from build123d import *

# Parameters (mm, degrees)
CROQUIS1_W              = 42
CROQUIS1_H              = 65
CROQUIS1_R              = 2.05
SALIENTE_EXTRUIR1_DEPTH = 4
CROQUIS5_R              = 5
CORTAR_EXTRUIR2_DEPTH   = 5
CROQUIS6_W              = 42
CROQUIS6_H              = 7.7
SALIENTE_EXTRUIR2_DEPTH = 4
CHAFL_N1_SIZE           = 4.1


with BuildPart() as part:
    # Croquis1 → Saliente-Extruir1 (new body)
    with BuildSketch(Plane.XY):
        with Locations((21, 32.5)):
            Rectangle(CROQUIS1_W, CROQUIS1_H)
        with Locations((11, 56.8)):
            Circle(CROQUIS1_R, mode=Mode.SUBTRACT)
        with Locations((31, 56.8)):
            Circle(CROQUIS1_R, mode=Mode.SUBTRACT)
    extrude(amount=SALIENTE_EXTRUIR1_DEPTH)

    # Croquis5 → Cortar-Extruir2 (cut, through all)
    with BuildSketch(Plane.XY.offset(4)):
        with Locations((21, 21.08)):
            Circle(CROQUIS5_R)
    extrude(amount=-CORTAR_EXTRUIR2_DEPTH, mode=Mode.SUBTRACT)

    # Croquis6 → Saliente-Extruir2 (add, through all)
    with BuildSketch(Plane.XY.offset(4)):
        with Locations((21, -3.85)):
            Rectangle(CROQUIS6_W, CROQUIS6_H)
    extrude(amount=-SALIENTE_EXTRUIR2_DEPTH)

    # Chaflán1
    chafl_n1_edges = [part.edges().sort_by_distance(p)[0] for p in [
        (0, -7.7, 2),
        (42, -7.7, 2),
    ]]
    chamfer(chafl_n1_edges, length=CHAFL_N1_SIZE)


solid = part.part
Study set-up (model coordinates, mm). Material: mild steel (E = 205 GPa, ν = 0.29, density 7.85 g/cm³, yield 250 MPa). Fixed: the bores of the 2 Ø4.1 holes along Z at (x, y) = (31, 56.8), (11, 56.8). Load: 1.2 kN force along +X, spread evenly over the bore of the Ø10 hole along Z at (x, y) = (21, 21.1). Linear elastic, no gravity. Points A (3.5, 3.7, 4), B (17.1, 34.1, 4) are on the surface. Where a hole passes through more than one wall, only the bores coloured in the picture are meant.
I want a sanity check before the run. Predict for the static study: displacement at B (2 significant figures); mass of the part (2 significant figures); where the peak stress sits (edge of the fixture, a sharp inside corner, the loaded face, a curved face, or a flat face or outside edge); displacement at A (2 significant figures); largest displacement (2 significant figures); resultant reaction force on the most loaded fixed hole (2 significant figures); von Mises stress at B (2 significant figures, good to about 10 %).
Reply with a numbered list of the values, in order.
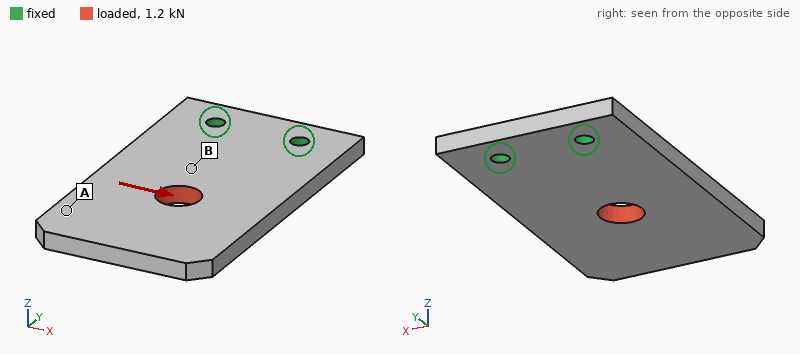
1. 6.4 µm
2. 92 g
3. edge of the fixture
4. 16 µm
5. 19 µm
6. 1.9 kN
7. 20 MPa
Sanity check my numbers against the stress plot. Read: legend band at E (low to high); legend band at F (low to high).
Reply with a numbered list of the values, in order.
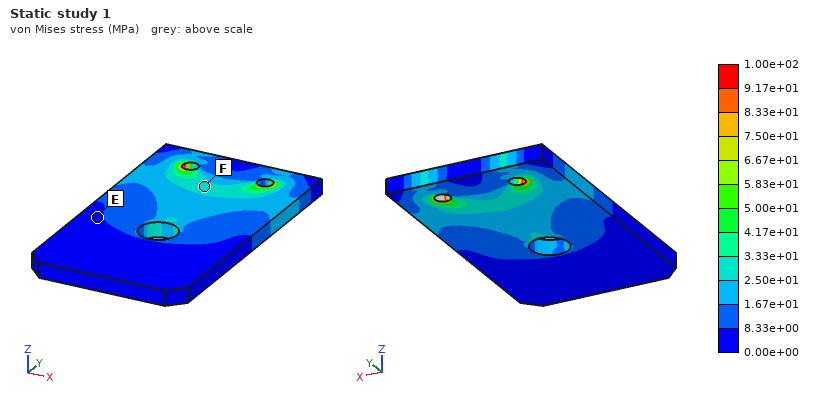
1. 0.00e+00 to 8.33e+00 MPa
2. 2.50e+01 to 3.33e+01 MPa
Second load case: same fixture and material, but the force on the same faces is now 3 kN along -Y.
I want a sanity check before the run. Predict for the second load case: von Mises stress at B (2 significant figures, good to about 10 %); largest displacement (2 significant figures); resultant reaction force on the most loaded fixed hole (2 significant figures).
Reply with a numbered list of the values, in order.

1. 24 MPa
2. 5.1 µm
3. 1.5 kN
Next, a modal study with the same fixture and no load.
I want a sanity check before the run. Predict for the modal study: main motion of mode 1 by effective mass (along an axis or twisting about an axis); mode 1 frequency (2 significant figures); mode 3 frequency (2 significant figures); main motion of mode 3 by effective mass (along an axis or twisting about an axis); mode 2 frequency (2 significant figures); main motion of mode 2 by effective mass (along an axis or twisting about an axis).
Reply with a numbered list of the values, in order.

1. along Z
2. 810 Hz
3. 4800 Hz
4. along Z
5. 2600 Hz
6. twisting about Y
